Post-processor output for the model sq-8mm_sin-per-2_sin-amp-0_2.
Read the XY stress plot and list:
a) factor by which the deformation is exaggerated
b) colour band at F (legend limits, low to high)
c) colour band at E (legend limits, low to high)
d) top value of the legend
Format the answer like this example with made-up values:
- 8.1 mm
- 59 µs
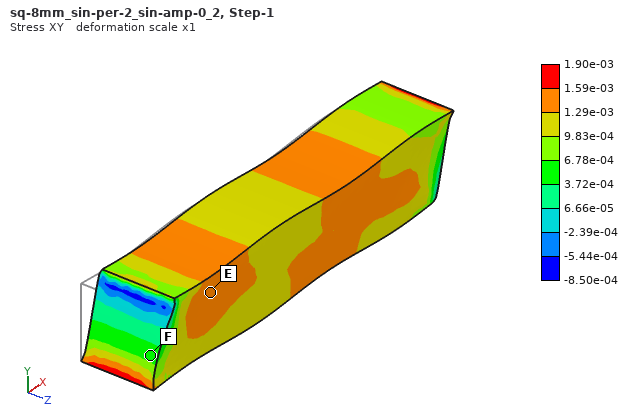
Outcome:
- 1
- 3.72e-04 to 6.78e-04
- 1.29e-03 to 1.59e-03
- 1.90e-03
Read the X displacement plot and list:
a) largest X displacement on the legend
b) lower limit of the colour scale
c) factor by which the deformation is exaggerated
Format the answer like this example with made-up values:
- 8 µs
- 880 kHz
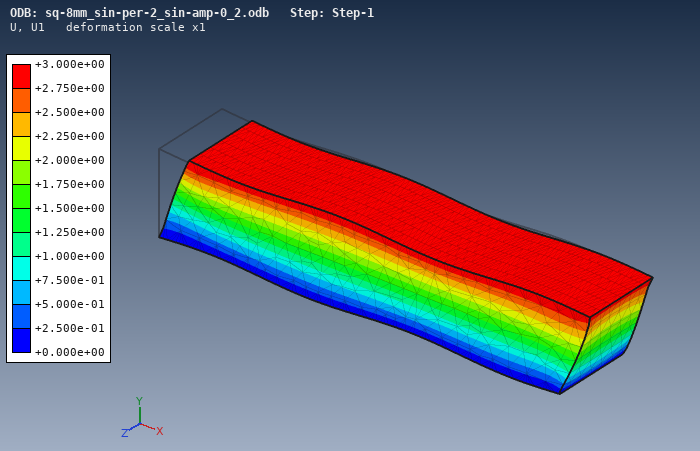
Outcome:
- +3.000e+00
- +0.000e+00
- 1
